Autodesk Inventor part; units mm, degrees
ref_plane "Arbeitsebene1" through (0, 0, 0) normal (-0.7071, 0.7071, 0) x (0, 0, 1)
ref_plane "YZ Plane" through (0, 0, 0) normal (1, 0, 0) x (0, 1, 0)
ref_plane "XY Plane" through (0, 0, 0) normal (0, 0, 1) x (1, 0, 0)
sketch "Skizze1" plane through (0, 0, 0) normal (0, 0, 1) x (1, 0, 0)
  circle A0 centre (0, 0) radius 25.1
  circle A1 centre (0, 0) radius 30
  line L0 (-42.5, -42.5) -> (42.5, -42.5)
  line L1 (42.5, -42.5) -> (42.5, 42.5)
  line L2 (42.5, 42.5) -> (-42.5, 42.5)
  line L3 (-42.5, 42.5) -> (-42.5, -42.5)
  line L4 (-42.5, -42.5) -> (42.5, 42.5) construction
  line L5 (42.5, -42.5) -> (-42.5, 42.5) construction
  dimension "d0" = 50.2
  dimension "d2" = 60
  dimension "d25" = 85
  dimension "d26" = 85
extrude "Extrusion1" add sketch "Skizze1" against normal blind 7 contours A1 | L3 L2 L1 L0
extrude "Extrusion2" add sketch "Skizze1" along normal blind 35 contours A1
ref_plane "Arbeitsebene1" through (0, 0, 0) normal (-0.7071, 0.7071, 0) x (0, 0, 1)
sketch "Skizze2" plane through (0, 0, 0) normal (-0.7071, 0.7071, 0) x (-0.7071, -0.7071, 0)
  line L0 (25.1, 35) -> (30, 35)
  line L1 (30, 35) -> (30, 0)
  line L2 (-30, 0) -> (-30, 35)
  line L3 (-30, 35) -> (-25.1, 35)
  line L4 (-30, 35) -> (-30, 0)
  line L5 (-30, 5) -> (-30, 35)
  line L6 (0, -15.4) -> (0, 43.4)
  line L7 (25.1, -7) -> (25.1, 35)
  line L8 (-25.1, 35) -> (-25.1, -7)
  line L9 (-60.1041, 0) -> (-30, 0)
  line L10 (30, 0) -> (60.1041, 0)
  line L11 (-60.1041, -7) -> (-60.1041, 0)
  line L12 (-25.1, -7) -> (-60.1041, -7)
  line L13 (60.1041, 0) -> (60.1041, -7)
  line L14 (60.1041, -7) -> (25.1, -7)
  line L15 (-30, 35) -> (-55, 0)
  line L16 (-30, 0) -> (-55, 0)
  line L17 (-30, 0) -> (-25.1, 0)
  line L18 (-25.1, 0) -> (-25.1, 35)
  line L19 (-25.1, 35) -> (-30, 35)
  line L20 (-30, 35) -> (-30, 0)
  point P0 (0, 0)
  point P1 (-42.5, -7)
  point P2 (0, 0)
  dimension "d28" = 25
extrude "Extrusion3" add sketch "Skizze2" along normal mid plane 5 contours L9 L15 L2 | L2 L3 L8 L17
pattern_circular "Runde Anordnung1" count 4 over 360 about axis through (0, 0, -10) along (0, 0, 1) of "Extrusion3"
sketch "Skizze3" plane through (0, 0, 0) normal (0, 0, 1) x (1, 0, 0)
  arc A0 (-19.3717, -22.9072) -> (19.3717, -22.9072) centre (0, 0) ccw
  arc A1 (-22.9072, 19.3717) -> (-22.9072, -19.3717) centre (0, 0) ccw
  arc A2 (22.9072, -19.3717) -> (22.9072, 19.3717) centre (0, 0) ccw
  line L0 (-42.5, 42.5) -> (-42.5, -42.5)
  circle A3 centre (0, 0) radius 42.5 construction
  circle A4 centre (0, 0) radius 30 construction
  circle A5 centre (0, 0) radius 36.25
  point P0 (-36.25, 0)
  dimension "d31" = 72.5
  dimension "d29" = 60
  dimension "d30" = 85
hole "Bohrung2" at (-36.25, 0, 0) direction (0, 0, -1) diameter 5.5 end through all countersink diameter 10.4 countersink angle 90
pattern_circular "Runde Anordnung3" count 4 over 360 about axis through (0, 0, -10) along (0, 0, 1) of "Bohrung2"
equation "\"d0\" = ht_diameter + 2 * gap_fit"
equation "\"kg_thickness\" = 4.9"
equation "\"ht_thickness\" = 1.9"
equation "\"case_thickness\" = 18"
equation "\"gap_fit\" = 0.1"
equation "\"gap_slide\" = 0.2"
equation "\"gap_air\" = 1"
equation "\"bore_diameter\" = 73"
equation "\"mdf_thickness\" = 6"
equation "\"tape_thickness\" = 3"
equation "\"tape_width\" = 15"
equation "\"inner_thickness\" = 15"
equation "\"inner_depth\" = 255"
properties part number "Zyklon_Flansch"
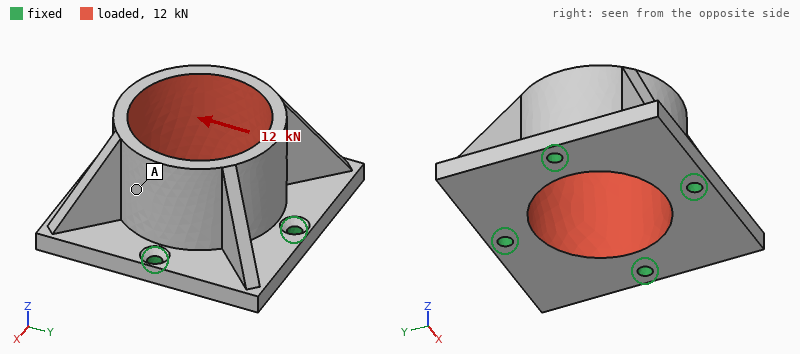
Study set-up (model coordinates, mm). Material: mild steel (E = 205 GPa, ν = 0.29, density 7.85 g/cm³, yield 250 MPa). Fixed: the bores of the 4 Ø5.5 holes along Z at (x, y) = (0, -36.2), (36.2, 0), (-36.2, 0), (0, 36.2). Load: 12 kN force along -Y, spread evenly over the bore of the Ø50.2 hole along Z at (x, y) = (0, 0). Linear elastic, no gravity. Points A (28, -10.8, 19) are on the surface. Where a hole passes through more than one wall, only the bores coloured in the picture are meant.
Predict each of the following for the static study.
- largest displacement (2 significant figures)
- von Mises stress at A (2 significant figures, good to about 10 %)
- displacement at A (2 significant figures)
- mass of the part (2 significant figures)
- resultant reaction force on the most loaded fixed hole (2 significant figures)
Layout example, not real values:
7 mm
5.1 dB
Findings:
16 µm
14 MPa
10.0 µm
580 g
4.2 kN
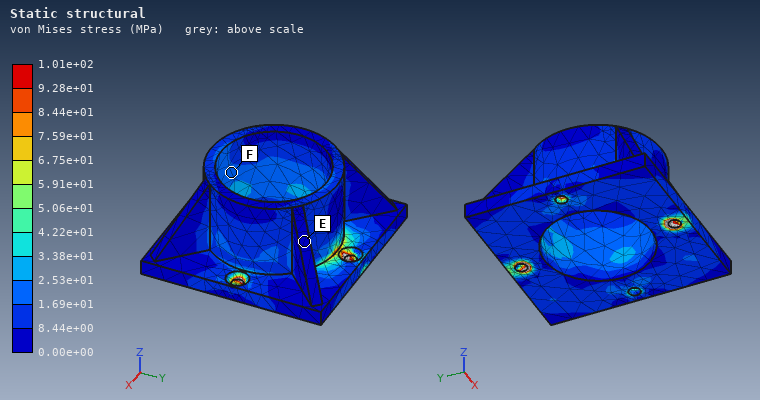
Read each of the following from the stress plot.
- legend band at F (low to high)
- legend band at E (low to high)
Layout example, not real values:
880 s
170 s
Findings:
1.69e+01 to 2.53e+01 MPa
0.00e+00 to 8.44e+00 MPa
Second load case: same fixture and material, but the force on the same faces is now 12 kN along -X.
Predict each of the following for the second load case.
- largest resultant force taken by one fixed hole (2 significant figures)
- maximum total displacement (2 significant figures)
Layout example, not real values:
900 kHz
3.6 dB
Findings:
4.2 kN
16 µm
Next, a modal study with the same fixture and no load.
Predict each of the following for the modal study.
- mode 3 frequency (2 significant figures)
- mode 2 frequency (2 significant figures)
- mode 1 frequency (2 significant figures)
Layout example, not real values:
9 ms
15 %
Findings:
6300 Hz
6300 Hz
4500 Hz
